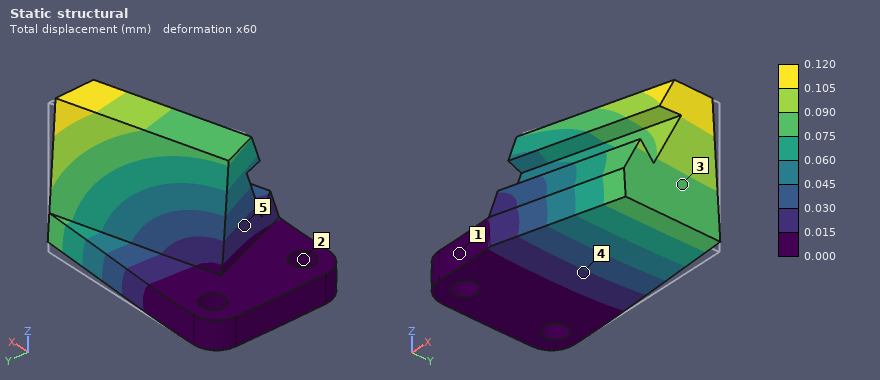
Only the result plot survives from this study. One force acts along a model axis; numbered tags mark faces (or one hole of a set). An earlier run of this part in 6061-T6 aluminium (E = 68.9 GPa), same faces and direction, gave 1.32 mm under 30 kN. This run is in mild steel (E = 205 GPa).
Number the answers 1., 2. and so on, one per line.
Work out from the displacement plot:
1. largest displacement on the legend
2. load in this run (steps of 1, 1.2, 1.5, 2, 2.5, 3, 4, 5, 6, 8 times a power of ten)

1. 0.120 mm
2. 8 kN
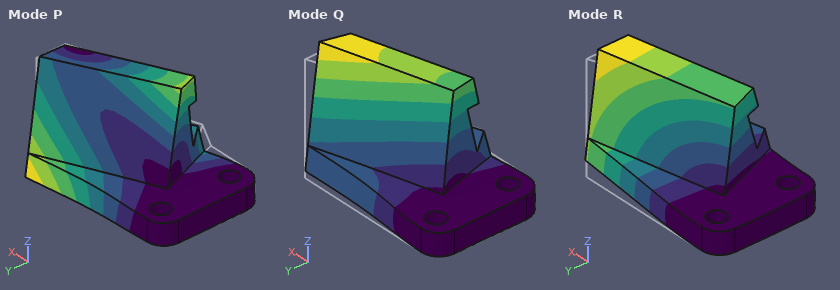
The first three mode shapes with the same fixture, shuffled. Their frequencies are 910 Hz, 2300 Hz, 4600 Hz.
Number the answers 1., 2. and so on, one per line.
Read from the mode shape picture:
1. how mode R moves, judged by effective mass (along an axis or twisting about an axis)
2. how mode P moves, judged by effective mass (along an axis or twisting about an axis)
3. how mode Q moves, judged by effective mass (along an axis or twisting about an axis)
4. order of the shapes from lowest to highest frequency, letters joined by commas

1. along Z
2. along Y
3. along Y
4. R, Q, P
